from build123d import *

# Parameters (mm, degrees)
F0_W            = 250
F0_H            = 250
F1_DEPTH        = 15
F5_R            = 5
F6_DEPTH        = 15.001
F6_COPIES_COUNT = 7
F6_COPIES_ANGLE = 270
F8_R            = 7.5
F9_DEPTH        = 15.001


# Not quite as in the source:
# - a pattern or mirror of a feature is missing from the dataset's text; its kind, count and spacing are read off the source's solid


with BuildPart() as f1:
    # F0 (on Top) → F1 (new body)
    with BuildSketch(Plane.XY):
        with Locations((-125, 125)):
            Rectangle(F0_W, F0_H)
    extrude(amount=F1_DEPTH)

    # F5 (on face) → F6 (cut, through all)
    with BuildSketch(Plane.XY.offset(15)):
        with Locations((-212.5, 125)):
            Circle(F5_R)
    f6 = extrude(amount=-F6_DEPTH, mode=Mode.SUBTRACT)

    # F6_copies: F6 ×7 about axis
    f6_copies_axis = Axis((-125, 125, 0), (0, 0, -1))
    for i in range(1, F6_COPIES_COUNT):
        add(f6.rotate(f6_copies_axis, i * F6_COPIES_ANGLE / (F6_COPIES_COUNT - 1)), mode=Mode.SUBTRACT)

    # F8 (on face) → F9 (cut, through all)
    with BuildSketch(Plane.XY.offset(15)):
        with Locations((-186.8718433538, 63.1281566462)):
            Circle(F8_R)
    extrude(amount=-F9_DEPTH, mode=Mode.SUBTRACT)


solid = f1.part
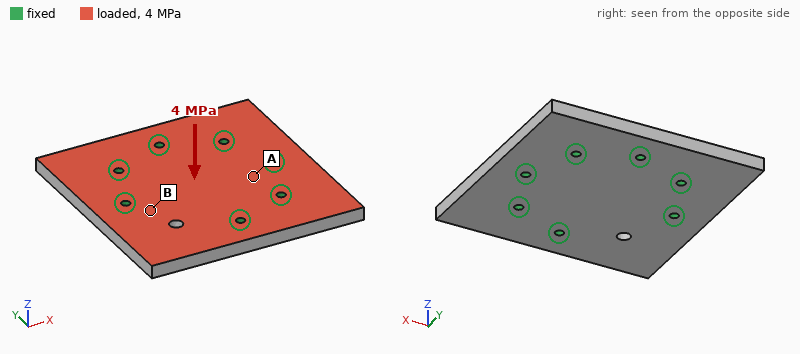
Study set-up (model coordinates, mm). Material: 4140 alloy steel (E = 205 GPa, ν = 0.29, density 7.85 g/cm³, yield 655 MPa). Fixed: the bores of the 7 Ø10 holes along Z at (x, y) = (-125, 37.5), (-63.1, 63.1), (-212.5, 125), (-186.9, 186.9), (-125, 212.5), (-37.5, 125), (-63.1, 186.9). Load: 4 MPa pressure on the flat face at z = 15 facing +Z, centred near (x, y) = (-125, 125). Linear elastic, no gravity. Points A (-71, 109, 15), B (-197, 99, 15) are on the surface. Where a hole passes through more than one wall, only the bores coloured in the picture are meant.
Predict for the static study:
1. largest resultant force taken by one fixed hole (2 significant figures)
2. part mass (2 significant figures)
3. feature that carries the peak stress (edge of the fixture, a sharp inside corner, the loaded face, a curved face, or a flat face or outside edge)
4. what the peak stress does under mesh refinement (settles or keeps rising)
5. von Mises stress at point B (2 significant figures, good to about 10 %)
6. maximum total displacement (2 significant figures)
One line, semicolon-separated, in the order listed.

48 kN; 7.3 kg; edge of the fixture; keeps rising; 180 MPa; 0.83 mm
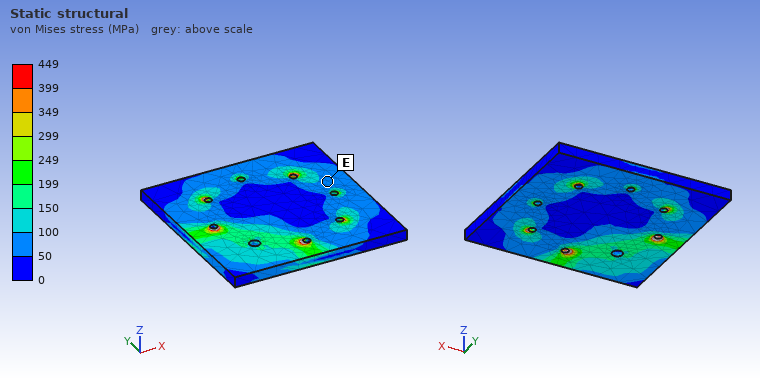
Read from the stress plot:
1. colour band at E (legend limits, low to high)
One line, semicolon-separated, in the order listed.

50 to 100 MPa
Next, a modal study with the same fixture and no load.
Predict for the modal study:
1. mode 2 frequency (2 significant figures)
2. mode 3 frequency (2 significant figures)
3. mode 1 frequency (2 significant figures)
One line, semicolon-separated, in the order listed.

2300 Hz; 2300 Hz; 1400 Hz
